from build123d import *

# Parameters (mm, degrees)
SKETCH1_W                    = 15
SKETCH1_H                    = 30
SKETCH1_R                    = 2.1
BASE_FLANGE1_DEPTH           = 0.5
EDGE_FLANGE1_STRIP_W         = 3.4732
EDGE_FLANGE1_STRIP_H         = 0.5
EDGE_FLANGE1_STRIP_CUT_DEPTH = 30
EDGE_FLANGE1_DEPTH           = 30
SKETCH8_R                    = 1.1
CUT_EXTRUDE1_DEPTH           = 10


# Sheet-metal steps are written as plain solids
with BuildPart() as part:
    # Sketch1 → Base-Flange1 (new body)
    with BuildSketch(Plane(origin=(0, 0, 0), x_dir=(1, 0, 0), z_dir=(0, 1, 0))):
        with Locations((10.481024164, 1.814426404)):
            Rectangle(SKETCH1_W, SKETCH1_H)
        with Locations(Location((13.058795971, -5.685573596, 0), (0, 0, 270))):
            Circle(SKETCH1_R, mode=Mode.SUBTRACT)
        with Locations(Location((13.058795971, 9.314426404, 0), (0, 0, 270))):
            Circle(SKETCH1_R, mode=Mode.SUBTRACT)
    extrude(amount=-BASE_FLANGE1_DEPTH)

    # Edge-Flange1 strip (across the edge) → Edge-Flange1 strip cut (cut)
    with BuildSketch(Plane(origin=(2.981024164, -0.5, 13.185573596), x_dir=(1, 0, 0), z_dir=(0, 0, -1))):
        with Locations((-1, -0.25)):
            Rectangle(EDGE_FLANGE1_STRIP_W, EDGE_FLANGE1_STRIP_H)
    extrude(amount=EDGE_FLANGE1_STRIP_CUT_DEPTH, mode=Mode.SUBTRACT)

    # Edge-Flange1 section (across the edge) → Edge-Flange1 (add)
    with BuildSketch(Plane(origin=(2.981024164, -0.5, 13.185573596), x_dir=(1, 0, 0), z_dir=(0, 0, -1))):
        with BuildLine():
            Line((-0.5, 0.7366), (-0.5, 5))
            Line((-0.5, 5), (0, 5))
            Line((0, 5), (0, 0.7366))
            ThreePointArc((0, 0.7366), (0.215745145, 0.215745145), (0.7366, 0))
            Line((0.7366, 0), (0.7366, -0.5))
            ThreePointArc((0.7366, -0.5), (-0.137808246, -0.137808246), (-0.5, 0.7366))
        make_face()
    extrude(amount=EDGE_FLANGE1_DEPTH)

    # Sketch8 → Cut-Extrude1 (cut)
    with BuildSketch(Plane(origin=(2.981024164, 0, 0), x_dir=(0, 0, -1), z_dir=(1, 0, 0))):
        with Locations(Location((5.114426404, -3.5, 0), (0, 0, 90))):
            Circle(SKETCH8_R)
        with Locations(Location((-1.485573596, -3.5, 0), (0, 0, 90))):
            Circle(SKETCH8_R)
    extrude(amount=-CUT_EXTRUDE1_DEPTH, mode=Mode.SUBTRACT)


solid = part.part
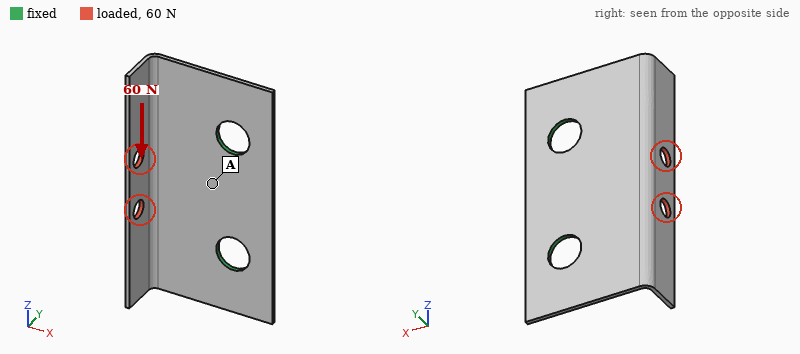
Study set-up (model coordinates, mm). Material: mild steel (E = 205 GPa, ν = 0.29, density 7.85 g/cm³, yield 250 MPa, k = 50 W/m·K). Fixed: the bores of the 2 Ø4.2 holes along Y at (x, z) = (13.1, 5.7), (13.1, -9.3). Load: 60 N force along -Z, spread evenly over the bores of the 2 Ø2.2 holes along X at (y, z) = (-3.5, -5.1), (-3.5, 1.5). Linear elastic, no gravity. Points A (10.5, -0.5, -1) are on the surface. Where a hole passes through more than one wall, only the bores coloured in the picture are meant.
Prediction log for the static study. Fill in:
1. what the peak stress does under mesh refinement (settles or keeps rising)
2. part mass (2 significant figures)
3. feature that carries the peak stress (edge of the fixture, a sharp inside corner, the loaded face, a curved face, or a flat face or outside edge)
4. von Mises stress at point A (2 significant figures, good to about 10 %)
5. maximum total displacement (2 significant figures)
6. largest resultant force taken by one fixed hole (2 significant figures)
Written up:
keeps rising
2.2 g
edge of the fixture
25 MPa
0.10 mm
44 N
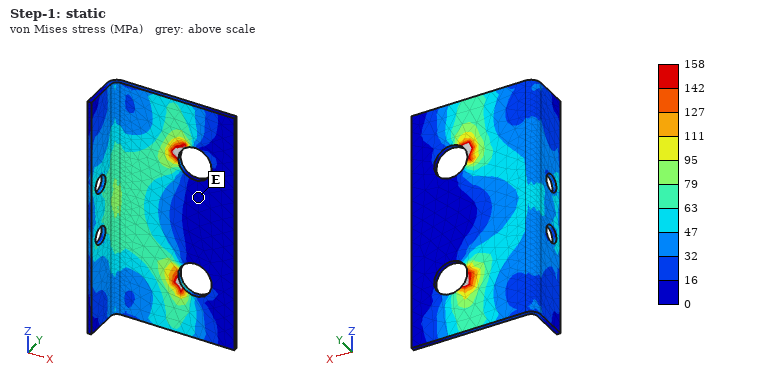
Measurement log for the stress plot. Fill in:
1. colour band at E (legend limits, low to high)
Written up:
0 to 16 MPa
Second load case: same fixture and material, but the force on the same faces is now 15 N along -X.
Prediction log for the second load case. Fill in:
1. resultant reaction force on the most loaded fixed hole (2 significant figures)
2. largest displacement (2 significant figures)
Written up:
8.0 N
55 µm
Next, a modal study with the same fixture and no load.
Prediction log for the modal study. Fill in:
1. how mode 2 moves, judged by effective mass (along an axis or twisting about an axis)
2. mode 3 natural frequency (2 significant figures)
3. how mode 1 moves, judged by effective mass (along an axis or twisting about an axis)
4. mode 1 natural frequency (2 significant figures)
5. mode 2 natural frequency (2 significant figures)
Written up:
twisting about X
9400 Hz
along Y
2600 Hz
3400 Hz
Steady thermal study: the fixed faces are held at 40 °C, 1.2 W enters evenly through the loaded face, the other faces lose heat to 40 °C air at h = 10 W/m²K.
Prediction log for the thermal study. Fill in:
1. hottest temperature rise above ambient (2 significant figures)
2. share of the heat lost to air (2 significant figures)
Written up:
31 K
8.7 %
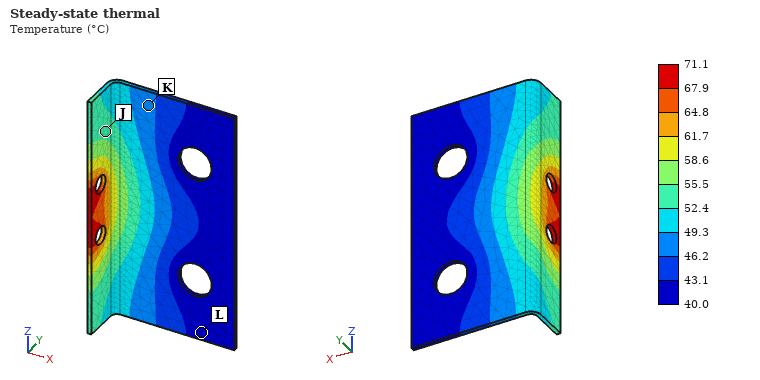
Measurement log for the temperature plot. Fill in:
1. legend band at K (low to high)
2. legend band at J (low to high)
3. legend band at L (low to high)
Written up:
46.2 to 49.3 °C
52.4 to 55.5 °C
40.0 to 43.1 °C
